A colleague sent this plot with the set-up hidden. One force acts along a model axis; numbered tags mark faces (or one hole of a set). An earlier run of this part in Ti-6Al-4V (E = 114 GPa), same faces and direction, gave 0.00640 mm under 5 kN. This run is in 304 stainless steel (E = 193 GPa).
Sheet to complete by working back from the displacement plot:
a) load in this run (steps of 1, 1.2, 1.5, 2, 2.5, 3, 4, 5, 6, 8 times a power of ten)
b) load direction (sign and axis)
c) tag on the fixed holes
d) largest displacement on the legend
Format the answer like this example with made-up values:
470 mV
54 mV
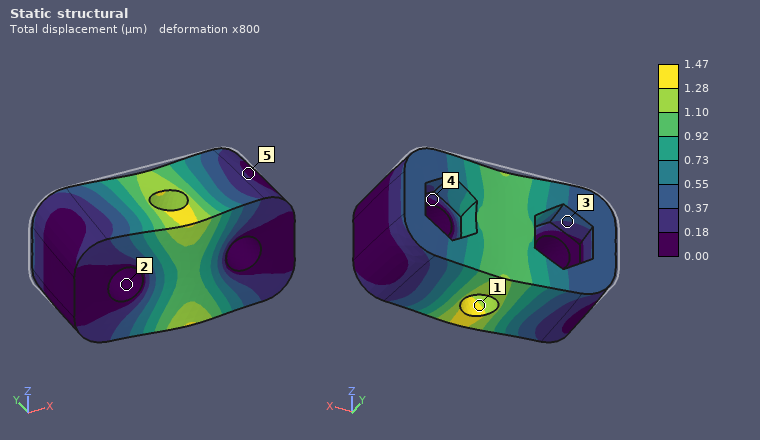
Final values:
2 kN
-Y
2
1.47 µm
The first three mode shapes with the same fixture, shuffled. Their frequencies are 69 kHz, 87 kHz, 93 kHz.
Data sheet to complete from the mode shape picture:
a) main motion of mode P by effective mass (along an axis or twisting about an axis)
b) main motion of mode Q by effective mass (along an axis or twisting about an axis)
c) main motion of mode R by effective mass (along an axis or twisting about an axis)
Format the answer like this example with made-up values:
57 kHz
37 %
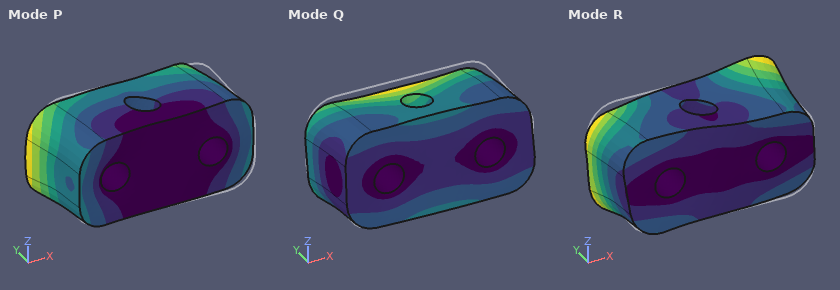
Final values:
along X
along Z
twisting about Y
